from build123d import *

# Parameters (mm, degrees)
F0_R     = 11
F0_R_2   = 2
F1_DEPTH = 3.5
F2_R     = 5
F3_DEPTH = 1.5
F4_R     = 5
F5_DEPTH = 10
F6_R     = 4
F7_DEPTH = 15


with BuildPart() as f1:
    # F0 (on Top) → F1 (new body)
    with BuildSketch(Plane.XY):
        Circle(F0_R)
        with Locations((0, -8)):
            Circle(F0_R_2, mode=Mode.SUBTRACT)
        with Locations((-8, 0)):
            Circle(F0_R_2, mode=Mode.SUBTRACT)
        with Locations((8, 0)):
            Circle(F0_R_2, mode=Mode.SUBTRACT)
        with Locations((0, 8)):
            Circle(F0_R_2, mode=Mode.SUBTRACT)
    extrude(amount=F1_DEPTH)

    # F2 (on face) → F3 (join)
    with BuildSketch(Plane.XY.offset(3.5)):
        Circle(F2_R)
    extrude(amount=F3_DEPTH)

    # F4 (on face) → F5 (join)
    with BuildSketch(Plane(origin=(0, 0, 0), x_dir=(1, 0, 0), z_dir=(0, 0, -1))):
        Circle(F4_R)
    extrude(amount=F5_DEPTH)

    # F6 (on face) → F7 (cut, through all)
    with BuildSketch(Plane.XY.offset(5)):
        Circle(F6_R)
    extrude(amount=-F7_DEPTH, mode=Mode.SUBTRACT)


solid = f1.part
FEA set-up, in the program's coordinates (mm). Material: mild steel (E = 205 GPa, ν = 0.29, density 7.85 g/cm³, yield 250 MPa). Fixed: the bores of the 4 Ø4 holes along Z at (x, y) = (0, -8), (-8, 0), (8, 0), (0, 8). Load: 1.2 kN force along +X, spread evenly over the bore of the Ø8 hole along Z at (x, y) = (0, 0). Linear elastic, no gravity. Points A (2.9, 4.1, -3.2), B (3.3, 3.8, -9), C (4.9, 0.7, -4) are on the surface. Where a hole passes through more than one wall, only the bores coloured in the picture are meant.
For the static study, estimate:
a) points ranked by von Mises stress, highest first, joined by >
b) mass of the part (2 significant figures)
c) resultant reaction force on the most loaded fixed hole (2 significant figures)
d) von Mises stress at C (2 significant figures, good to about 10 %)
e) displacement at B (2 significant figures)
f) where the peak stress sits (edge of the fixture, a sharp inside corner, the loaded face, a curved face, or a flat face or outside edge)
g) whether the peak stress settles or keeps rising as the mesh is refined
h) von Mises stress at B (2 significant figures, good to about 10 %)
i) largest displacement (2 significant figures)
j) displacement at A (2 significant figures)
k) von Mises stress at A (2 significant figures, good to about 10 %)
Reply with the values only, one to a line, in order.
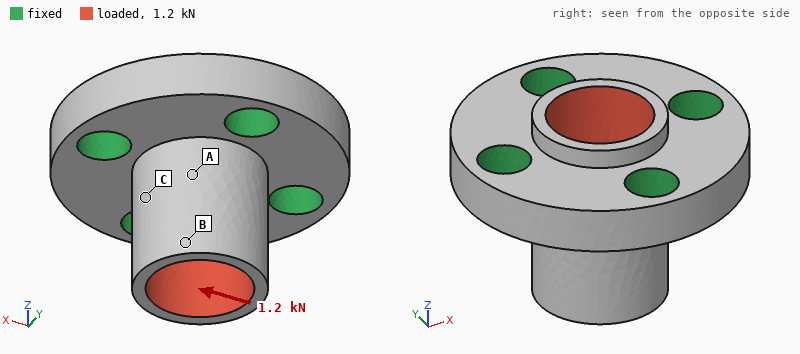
A > C > B
10 g
510 N
24 MPa
6.7 µm
a sharp inside corner
keeps rising
12 MPa
7.5 µm
3.2 µm
48 MPa
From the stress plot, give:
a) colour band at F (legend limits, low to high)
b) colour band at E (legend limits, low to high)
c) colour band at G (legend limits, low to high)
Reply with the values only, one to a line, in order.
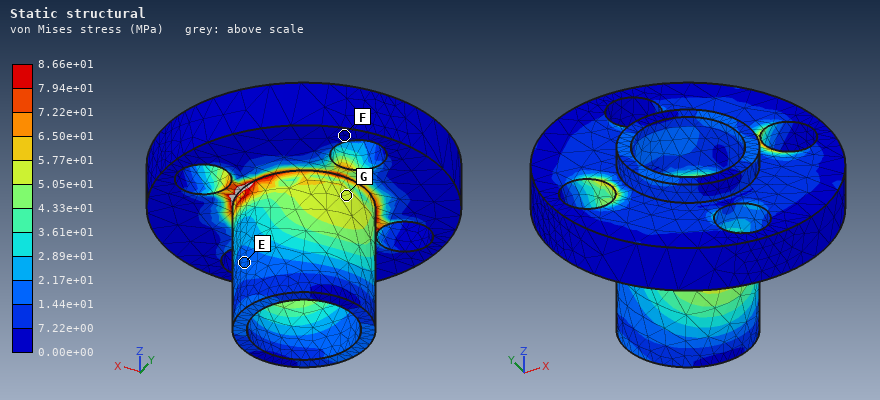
0.00e+00 to 7.22e+00 MPa
1.44e+01 to 2.17e+01 MPa
5.05e+01 to 5.77e+01 MPa
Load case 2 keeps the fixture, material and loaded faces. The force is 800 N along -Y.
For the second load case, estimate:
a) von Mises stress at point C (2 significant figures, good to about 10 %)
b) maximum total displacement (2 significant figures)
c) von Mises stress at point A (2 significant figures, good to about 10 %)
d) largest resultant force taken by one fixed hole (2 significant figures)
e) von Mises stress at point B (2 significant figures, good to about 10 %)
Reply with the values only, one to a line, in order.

35 MPa
5.0 µm
25 MPa
340 N
8.2 MPa
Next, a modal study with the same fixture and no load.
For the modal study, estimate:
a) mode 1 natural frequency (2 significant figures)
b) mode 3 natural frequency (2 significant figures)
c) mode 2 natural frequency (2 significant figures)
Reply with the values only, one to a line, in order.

40 kHz
41 kHz
41 kHz
